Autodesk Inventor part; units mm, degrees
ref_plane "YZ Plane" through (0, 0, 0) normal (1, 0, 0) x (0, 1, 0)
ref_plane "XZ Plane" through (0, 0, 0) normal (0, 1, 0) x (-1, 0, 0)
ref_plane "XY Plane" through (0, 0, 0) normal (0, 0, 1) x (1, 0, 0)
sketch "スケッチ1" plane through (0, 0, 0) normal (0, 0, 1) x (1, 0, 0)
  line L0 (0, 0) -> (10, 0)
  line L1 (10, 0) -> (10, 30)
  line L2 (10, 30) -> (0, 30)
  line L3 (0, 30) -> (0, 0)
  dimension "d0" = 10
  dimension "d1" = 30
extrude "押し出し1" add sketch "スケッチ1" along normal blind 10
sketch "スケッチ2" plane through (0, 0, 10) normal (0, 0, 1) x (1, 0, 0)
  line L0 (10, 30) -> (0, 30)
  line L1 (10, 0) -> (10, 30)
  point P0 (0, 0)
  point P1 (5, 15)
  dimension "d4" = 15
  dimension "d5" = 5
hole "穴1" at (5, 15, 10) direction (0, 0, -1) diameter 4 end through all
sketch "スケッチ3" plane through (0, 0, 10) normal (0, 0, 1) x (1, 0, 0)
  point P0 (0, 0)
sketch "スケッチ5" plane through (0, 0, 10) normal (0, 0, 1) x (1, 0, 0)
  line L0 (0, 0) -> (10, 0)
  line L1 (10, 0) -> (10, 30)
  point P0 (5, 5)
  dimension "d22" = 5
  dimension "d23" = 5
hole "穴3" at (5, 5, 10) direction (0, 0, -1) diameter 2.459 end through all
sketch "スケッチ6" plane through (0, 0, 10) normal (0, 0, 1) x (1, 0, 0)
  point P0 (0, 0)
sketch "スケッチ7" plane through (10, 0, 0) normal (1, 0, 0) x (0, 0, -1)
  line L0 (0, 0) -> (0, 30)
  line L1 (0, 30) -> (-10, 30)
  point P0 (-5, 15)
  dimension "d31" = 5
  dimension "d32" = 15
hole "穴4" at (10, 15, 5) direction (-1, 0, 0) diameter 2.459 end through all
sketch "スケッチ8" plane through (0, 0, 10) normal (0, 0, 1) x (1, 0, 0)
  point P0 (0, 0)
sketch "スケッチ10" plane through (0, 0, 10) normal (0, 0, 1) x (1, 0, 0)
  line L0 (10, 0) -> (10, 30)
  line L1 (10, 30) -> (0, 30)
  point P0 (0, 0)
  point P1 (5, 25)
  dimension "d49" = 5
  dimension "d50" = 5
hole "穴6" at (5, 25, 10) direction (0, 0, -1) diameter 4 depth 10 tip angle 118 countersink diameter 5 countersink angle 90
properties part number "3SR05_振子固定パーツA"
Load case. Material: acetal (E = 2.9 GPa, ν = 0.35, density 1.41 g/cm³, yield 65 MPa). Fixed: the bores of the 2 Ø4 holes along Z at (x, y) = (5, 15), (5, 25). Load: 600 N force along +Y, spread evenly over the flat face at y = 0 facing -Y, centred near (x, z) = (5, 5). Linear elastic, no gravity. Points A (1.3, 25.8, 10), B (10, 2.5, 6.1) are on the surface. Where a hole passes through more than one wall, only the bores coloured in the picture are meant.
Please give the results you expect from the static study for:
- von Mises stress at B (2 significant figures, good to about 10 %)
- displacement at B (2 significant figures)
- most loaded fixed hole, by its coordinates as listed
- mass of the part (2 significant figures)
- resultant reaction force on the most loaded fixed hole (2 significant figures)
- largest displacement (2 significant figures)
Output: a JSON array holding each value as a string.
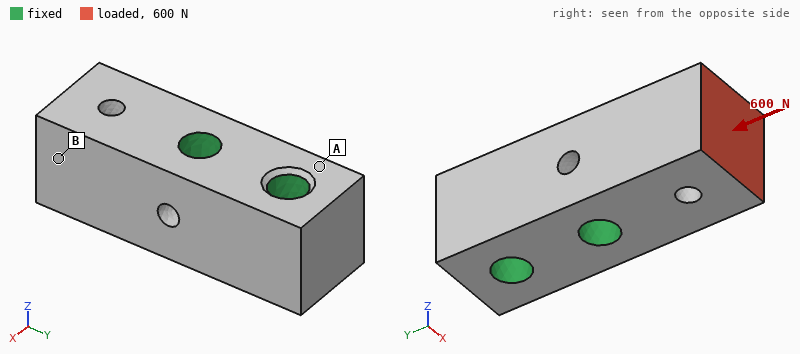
["5.9 MPa", "27 µm", "(5, 15)", "3.8 g", "550 N", "37 µm"]
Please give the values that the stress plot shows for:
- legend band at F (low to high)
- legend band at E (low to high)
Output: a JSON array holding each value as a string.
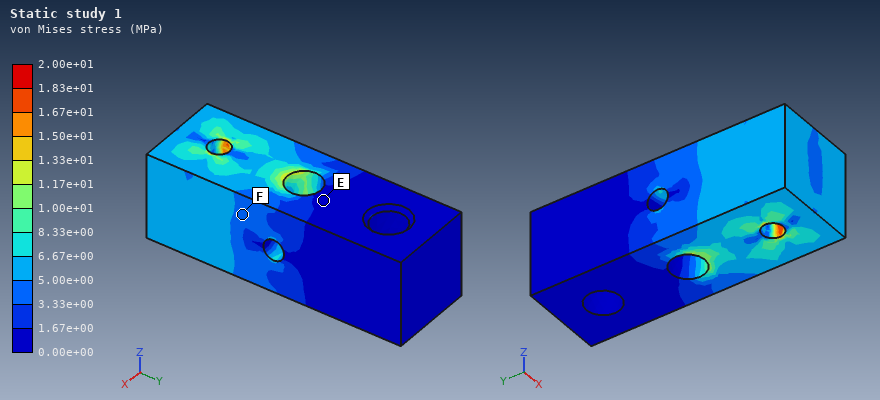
["3.33e+00 to 5.00e+00 MPa", "0.00e+00 to 1.67e+00 MPa"]
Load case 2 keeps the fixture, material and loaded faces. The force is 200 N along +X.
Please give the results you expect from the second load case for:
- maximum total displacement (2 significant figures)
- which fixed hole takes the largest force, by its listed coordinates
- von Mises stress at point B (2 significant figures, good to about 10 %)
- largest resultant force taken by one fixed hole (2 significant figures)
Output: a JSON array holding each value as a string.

["0.18 mm", "(5, 15)", "2.9 MPa", "290 N"]
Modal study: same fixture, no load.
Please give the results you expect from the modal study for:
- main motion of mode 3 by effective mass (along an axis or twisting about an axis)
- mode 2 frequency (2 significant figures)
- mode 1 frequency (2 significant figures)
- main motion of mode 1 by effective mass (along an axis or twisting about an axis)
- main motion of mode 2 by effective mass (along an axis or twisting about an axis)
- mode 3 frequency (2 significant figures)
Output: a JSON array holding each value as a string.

["twisting about Y", "8700 Hz", "7000 Hz", "along X", "along Z", "14 kHz"]
